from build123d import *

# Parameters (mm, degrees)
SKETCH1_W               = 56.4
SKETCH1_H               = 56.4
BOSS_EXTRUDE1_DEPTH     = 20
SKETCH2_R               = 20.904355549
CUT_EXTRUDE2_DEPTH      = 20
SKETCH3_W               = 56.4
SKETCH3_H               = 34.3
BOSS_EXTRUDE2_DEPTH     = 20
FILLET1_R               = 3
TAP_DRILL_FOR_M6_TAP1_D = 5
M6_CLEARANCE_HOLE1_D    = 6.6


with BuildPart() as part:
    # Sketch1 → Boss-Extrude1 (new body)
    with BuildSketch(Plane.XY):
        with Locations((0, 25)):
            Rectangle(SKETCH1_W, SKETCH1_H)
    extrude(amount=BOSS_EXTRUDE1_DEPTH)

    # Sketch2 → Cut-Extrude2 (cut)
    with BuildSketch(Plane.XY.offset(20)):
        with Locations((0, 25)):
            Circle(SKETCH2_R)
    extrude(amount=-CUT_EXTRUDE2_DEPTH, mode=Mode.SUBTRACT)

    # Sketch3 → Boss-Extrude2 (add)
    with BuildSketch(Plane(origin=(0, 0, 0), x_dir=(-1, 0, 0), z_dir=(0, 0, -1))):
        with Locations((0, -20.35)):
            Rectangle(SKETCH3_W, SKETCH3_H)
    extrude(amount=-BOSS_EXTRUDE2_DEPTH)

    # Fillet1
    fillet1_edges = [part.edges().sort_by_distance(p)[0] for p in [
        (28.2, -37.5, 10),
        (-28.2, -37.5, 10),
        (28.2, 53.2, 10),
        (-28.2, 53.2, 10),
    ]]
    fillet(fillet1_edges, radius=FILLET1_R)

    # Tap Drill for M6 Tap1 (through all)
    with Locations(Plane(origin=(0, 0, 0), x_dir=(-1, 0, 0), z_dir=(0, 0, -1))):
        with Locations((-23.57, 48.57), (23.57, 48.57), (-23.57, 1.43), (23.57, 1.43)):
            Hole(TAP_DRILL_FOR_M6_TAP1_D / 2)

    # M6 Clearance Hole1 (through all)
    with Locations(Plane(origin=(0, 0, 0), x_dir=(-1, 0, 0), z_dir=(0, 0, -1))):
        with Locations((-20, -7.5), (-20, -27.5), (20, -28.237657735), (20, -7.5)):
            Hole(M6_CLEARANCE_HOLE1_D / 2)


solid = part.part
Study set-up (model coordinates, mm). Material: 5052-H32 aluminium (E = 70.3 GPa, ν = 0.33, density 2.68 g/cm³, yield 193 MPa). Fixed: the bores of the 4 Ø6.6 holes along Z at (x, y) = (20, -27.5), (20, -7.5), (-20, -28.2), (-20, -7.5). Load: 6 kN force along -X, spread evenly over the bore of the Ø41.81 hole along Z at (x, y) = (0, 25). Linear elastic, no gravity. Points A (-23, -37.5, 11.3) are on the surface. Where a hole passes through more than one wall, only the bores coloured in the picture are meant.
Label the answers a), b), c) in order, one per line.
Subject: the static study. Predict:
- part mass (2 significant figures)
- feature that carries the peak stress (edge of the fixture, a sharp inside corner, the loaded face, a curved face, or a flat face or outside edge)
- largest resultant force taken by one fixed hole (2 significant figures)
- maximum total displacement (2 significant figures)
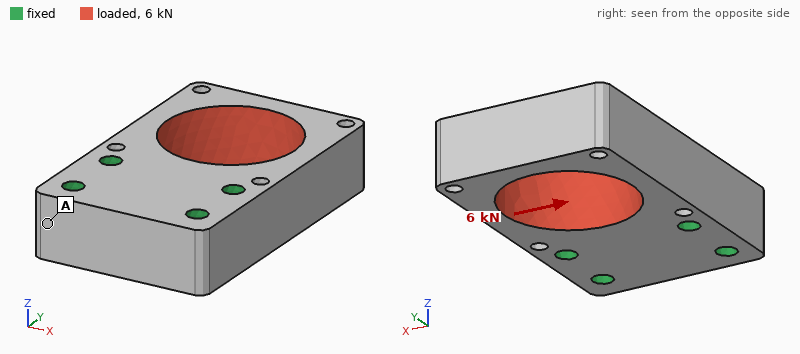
a) 190 g
b) a curved face
c) 4.6 kN
d) 0.11 mm
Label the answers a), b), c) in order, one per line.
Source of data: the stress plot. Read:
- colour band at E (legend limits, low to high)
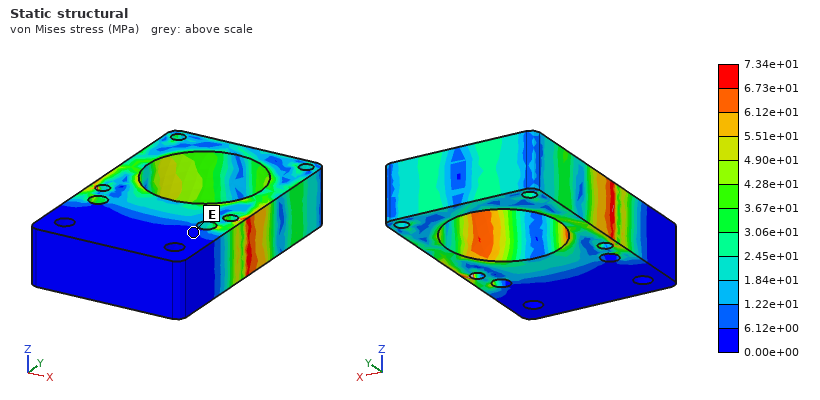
a) 0.00e+00 to 6.12e+00 MPa
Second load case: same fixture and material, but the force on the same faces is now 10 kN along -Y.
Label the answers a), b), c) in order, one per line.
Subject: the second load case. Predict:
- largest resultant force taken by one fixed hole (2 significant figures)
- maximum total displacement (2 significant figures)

a) 4.5 kN
b) 39 µm
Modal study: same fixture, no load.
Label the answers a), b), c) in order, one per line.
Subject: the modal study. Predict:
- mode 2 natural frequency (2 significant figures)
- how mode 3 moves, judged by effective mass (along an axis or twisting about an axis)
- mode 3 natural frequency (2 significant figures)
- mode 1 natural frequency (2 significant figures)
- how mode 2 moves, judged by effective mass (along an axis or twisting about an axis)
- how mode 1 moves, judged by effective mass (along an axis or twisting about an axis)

a) 4200 Hz
b) twisting about Y
c) 6100 Hz
d) 3300 Hz
e) along X
f) along Z
